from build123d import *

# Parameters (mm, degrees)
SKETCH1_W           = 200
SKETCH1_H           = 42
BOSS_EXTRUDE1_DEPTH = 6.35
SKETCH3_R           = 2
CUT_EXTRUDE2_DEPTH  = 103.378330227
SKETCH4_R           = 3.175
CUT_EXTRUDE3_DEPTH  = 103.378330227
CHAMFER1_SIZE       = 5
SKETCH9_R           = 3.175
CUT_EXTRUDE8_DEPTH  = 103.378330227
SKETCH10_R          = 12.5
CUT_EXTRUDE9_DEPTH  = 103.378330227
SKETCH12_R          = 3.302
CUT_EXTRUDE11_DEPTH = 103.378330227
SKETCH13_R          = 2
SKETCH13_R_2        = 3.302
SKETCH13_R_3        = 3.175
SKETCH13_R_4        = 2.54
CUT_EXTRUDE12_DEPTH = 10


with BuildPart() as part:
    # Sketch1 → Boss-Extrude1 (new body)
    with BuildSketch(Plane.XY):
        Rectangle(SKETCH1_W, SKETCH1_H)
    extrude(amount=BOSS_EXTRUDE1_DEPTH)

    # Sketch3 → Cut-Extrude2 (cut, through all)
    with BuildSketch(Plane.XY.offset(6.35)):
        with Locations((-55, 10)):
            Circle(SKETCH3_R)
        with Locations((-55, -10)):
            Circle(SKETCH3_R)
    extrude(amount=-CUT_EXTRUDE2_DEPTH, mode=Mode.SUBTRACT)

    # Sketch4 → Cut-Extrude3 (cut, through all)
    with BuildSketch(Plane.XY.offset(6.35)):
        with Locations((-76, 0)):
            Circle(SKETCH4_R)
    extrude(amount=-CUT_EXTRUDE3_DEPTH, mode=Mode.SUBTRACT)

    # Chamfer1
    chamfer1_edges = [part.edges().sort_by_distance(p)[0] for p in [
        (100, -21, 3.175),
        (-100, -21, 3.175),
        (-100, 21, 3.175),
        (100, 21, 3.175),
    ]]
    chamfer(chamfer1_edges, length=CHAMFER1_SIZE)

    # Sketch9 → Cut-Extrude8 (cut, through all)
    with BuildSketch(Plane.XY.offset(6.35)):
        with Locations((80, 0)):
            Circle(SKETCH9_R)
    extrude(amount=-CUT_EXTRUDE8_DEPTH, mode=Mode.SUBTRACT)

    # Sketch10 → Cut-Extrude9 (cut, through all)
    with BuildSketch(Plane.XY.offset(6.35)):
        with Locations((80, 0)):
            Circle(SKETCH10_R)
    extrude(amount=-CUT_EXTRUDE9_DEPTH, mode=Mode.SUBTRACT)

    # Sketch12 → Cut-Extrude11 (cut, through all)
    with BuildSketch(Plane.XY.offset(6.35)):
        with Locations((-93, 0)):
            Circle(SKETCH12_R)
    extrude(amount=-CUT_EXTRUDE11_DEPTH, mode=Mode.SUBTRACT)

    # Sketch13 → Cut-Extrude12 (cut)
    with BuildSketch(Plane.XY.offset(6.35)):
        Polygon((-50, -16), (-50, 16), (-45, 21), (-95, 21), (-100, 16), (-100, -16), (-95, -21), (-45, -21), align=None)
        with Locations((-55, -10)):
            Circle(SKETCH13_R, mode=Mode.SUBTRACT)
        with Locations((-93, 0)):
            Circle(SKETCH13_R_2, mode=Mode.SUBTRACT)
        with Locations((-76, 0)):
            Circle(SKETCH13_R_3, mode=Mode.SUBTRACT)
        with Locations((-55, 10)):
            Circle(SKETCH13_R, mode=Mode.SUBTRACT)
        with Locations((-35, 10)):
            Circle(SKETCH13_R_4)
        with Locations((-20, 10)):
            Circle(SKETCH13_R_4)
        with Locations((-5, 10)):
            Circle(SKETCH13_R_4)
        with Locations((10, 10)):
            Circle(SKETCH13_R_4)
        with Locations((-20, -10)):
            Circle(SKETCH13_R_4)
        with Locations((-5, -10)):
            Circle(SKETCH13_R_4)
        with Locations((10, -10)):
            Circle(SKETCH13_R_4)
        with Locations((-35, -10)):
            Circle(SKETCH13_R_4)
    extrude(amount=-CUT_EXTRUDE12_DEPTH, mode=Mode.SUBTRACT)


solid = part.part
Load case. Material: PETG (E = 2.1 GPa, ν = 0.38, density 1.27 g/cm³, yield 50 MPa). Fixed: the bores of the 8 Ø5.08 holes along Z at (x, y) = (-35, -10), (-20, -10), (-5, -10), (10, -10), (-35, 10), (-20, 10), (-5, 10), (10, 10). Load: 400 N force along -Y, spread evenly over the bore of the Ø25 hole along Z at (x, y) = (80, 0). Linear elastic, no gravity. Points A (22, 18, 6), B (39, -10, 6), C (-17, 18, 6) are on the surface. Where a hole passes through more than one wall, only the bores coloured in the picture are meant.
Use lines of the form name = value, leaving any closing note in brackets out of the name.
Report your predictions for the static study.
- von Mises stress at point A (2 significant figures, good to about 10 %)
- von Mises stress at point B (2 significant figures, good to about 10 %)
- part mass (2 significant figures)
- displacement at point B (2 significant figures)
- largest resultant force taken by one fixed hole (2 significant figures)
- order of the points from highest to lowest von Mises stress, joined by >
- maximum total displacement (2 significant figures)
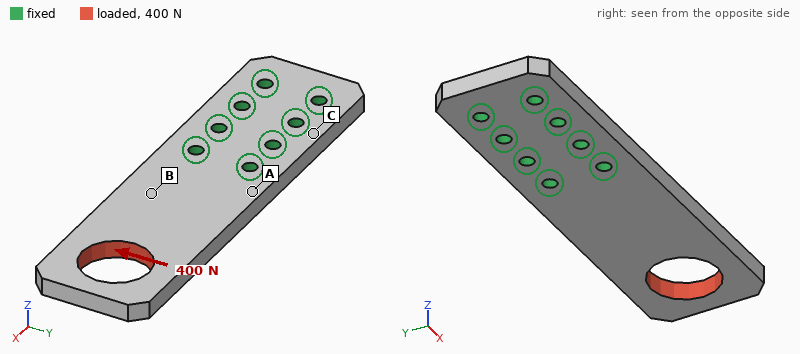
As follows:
von Mises stress at point A = 9.7 MPa
von Mises stress at point B = 5.0 MPa
part mass = 45 g
displacement at point B = 0.26 mm
largest resultant force taken by one fixed hole = 870 N
order of the points from highest to lowest von Mises stress, joined by > = A > B > C
maximum total displacement = 1.3 mm
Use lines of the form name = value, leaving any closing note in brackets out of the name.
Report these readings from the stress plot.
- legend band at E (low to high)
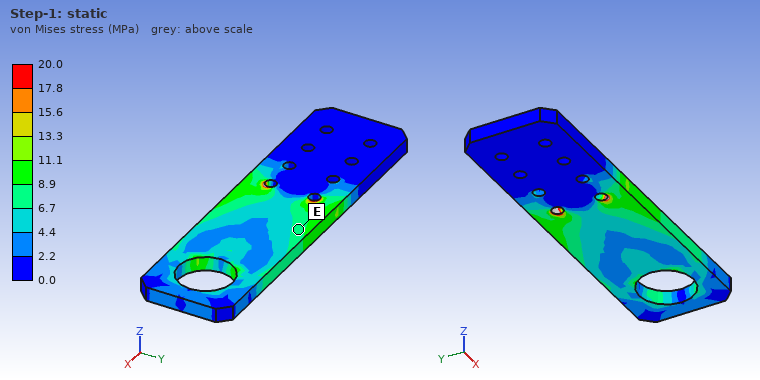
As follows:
legend band at E = 6.7 to 8.9 MPa
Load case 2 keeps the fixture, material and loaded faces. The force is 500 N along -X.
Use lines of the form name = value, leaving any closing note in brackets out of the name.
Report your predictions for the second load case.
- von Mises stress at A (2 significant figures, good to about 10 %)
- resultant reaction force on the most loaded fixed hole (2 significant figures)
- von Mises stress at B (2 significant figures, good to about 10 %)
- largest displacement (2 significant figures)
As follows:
von Mises stress at A = 1.6 MPa
resultant reaction force on the most loaded fixed hole = 210 N
von Mises stress at B = 1.8 MPa
largest displacement = 0.14 mm
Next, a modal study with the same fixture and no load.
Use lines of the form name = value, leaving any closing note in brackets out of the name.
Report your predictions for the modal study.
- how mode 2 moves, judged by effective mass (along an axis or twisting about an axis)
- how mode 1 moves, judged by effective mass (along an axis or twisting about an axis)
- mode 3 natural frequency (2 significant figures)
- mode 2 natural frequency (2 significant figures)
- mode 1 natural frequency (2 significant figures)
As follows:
how mode 2 moves, judged by effective mass = twisting about X
how mode 1 moves, judged by effective mass = along Z
mode 3 natural frequency = 940 Hz
mode 2 natural frequency = 690 Hz
mode 1 natural frequency = 200 Hz
